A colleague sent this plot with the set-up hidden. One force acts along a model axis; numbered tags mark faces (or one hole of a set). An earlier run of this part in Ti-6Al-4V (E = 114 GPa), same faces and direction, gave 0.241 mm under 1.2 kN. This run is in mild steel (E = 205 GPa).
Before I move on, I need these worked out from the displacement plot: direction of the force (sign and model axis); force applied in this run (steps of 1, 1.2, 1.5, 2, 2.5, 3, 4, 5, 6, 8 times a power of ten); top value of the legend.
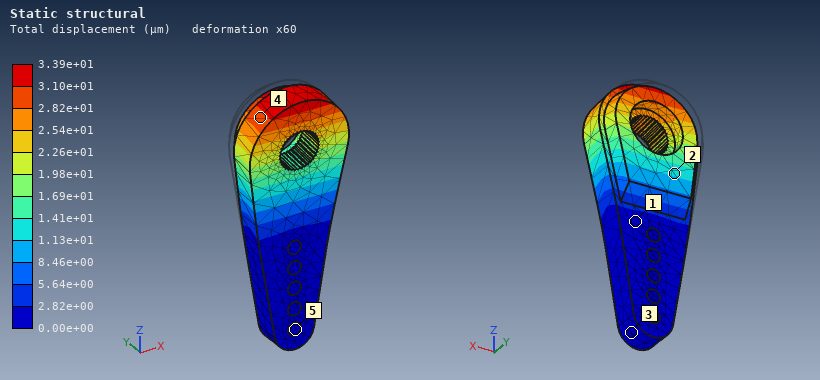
-Y
300 N
3.39e+01 µm
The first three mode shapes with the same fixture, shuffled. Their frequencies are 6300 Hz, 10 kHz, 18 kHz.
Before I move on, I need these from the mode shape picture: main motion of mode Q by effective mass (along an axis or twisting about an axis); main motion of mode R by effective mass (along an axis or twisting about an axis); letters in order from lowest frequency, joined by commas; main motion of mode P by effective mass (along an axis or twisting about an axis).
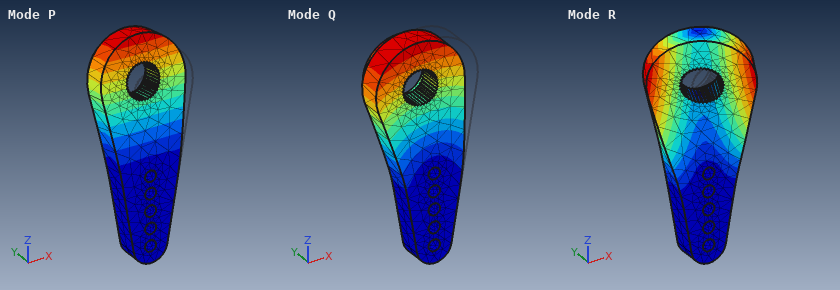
along X
twisting about Z
P, Q, R
along Y
